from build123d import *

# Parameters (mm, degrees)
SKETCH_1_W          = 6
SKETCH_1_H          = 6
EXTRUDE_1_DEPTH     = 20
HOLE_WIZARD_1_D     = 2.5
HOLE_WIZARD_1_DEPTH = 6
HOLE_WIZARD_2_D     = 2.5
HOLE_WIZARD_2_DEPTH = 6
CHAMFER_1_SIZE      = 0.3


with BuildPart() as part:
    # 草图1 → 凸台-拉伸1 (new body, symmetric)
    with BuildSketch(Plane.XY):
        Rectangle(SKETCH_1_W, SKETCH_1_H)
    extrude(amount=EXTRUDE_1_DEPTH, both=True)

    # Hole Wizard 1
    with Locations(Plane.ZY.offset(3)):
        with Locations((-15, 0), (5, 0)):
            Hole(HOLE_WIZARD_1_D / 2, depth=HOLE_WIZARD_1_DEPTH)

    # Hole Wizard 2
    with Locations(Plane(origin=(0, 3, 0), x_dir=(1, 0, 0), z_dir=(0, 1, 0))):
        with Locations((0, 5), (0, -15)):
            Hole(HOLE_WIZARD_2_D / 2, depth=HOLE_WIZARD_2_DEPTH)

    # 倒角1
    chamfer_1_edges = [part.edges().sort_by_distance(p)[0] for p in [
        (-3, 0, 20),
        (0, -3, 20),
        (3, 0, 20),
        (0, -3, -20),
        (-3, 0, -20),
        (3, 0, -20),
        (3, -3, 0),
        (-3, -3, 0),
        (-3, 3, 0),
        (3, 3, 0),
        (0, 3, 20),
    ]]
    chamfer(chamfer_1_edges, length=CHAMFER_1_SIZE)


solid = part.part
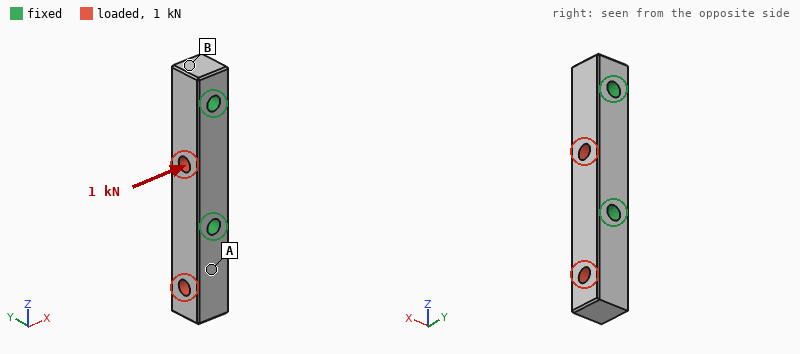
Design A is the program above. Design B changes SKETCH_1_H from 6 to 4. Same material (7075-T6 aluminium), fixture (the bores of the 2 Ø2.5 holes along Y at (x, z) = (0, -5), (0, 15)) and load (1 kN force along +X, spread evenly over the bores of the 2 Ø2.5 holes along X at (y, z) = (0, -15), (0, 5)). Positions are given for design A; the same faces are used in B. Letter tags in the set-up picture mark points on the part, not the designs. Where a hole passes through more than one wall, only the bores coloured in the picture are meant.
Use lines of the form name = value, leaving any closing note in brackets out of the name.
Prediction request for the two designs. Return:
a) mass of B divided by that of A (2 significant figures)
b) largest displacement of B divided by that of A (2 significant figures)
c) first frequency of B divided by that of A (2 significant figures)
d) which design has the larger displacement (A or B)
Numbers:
mass of B divided by that of A = 0.65
largest displacement of B divided by that of A = 1.5
first frequency of B divided by that of A = 0.83
which design has the larger displacement = B
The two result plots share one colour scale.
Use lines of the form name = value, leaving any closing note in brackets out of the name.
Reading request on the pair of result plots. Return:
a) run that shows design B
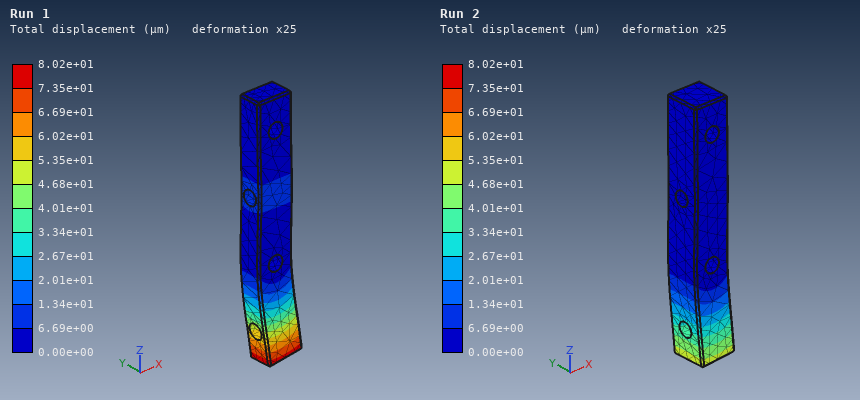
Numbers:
run that shows design B = Run 1
